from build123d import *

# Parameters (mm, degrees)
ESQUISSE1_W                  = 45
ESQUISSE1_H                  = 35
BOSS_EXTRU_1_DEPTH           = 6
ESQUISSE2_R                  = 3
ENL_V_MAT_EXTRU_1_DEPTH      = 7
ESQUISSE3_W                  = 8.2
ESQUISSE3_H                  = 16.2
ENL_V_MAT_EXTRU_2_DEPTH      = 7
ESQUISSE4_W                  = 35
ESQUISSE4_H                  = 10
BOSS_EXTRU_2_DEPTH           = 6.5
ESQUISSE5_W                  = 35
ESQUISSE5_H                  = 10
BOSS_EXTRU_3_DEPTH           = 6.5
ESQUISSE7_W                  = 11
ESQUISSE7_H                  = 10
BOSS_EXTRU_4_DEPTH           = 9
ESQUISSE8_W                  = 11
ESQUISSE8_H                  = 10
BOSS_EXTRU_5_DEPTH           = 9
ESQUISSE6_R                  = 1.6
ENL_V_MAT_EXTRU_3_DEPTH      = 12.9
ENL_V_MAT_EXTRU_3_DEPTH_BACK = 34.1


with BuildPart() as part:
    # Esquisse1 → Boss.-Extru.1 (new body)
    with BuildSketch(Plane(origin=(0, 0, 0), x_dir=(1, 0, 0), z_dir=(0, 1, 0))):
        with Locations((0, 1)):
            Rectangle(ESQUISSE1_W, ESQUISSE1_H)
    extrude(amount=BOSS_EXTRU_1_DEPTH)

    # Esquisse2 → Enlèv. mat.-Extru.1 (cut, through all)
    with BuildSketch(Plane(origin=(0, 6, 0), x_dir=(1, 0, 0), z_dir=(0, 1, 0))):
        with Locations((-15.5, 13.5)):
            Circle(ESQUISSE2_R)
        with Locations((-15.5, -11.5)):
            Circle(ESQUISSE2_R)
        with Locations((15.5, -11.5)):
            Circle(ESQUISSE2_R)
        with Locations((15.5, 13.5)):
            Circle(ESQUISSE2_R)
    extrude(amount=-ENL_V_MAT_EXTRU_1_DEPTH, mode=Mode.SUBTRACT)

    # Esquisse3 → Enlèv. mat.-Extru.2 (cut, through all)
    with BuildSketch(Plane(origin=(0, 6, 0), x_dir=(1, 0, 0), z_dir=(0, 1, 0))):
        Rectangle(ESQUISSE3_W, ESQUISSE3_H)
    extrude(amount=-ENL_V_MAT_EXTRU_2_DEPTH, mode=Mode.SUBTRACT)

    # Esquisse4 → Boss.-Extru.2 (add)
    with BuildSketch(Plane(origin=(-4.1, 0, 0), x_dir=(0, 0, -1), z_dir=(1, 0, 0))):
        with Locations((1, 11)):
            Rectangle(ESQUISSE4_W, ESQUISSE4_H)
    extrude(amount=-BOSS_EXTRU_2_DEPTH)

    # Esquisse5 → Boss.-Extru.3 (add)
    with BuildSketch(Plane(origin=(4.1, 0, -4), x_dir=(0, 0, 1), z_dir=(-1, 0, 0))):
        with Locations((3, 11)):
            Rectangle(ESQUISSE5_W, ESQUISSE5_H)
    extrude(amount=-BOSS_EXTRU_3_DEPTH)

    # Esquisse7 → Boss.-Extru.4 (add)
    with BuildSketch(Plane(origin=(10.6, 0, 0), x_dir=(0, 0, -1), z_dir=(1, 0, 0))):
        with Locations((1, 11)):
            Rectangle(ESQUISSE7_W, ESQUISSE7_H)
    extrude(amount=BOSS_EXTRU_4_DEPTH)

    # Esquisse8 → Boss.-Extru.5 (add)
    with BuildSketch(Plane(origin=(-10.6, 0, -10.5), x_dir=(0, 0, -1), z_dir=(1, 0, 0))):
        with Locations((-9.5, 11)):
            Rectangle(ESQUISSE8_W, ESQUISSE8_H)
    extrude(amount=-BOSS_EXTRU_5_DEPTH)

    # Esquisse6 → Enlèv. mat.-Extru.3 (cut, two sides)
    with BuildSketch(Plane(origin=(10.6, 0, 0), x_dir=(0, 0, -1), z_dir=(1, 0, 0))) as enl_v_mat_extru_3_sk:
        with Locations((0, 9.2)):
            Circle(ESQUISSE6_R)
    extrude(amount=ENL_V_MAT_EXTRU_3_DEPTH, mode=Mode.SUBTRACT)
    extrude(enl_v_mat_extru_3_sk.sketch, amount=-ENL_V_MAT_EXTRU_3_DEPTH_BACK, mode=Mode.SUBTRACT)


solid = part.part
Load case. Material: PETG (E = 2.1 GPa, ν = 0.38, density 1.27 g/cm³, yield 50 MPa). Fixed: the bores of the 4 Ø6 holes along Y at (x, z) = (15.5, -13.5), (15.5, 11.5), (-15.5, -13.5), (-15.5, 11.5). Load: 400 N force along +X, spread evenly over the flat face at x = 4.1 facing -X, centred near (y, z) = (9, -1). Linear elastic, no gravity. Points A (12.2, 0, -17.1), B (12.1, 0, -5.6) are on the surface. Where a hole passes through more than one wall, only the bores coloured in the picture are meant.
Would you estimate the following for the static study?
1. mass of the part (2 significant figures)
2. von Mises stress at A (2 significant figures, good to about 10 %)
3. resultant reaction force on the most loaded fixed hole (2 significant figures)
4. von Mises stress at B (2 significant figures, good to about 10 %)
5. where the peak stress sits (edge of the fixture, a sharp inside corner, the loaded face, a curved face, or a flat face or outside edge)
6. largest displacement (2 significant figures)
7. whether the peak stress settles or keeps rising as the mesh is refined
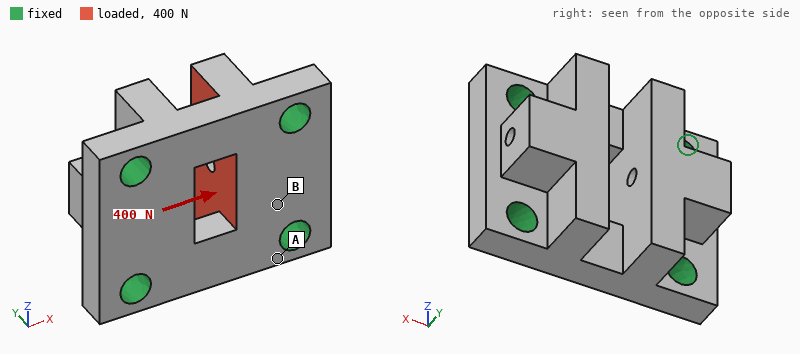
18 g
2.3 MPa
180 N
0.82 MPa
edge of the fixture
91 µm
keeps rising
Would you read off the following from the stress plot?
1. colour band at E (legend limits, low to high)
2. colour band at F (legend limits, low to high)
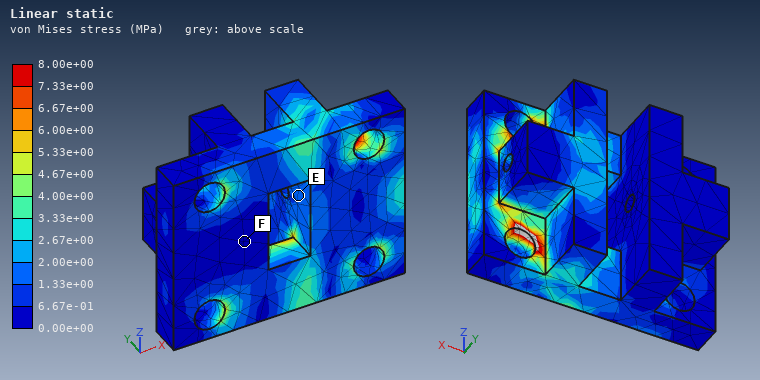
1.33e+00 to 2.00e+00 MPa
0.00e+00 to 6.67e-01 MPa
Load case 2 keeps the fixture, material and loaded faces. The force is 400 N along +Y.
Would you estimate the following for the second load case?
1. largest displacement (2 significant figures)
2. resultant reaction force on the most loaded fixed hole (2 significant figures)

0.12 mm
160 N
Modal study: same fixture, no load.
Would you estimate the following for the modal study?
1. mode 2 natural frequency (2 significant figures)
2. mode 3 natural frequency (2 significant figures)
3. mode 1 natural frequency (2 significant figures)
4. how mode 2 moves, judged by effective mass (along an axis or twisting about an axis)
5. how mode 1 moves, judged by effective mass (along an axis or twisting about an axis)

6300 Hz
6800 Hz
4300 Hz
along X
along Y
